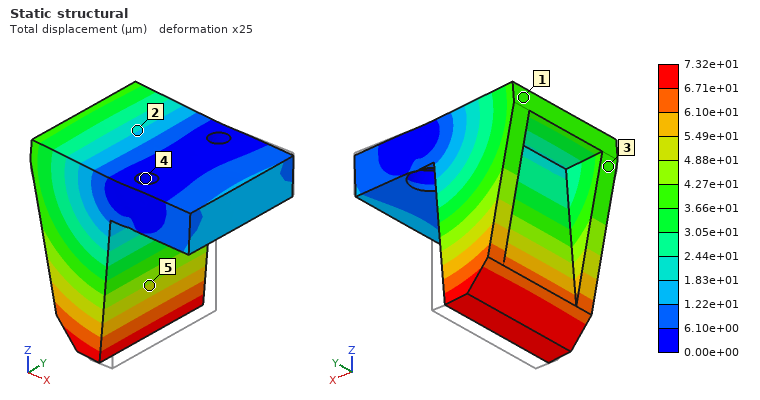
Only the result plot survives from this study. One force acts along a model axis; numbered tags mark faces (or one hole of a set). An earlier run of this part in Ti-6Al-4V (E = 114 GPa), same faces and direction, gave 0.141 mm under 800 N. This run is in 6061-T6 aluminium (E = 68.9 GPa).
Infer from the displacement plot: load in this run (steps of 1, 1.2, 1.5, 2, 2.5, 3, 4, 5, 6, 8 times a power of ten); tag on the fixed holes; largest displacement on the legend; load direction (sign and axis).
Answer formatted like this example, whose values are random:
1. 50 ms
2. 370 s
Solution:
1. 250 N
2. 4
3. 7.32e+01 µm
4. -X
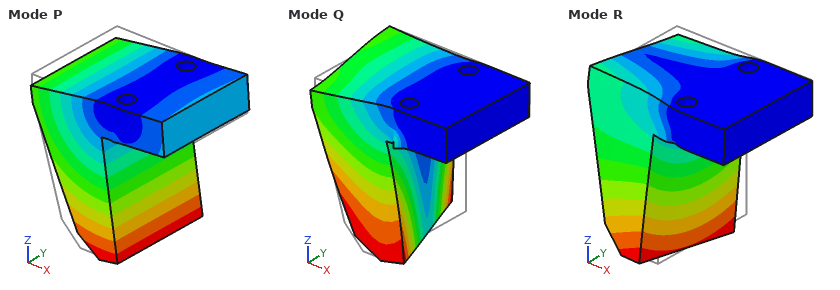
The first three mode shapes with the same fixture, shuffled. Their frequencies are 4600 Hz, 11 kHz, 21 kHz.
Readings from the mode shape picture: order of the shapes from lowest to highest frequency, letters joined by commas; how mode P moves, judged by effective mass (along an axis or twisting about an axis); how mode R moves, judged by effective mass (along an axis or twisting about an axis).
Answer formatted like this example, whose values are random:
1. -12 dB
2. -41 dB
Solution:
1. P, R, Q
2. along X
3. along Y
